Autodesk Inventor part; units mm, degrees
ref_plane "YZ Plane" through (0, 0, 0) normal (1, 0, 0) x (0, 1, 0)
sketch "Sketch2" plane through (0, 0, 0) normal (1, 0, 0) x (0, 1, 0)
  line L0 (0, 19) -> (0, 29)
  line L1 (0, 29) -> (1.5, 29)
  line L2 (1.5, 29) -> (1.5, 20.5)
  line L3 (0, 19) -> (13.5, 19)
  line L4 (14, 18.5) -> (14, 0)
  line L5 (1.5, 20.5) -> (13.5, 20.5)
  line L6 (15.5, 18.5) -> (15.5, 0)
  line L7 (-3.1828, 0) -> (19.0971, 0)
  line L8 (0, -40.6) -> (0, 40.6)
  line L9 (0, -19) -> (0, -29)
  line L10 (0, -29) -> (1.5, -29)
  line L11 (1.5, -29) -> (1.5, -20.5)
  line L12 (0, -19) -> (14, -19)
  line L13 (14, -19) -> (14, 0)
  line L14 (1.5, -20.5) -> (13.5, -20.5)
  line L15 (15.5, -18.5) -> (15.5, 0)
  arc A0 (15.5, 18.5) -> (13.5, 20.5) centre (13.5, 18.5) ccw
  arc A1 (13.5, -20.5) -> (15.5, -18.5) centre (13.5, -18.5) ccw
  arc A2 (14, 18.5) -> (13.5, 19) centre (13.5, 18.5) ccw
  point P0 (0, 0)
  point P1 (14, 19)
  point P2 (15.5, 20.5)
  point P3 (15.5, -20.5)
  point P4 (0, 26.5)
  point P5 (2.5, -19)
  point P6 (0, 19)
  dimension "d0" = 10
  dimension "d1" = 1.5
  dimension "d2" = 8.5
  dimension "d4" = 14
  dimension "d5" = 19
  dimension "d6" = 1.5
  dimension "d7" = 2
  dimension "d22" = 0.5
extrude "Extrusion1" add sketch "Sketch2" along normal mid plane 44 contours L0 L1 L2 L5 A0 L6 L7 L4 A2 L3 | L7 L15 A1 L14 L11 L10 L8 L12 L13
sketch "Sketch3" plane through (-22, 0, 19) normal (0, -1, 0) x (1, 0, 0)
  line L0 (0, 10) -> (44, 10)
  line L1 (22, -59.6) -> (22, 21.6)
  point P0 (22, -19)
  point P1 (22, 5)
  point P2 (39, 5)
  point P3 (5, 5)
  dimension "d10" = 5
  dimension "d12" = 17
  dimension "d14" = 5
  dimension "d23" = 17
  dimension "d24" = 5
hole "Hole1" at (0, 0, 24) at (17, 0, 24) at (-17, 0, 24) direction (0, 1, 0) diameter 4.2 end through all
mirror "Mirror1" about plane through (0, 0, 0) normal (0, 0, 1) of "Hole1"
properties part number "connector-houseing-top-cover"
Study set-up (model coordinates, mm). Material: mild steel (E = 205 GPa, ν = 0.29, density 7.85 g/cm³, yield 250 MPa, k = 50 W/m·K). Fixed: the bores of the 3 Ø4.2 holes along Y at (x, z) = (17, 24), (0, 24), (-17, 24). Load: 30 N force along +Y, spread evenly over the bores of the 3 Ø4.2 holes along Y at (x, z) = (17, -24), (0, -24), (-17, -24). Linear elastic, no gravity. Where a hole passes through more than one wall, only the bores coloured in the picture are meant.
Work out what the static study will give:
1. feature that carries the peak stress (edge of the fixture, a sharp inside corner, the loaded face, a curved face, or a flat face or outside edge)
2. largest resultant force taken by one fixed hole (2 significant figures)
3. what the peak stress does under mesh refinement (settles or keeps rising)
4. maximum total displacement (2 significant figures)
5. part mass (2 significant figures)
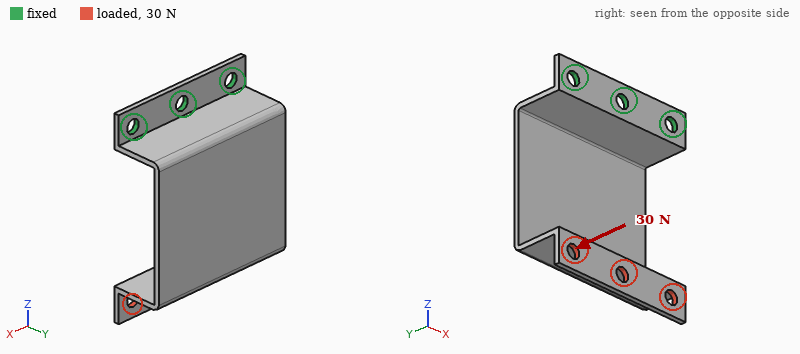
edge of the fixture
17 N
keeps rising
0.78 mm
43 g
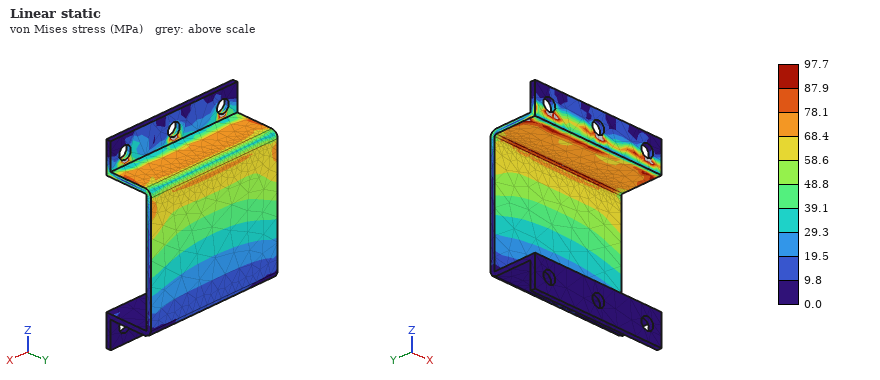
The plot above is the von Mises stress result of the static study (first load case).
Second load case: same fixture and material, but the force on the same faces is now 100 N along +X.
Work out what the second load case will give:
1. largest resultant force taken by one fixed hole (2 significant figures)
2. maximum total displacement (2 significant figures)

130 N
0.60 mm
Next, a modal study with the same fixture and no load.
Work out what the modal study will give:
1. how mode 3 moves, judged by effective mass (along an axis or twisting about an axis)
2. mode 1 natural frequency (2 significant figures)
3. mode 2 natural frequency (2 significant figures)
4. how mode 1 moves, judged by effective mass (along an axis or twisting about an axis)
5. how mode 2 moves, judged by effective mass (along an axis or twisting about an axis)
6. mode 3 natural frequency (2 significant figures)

along Z
280 Hz
630 Hz
along Y
along X
1100 Hz
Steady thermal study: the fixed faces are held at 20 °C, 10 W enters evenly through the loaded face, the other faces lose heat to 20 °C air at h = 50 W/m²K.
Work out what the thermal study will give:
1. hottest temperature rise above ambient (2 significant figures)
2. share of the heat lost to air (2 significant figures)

77 K
89 %
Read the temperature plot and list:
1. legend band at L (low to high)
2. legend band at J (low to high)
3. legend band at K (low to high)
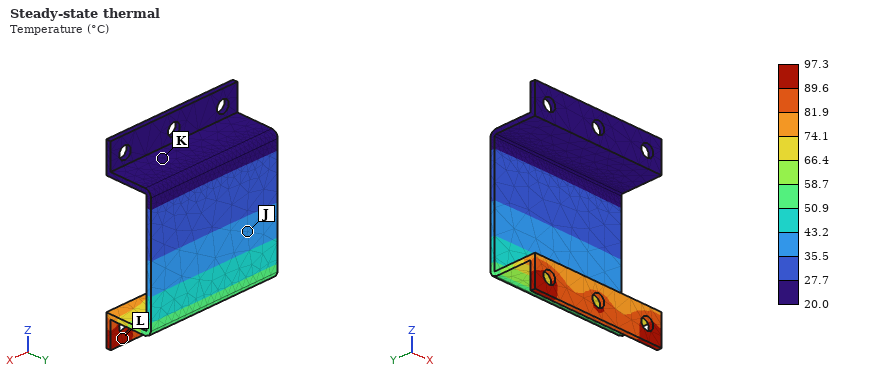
89.6 to 97.3 °C
35.5 to 43.2 °C
20.0 to 27.7 °C
